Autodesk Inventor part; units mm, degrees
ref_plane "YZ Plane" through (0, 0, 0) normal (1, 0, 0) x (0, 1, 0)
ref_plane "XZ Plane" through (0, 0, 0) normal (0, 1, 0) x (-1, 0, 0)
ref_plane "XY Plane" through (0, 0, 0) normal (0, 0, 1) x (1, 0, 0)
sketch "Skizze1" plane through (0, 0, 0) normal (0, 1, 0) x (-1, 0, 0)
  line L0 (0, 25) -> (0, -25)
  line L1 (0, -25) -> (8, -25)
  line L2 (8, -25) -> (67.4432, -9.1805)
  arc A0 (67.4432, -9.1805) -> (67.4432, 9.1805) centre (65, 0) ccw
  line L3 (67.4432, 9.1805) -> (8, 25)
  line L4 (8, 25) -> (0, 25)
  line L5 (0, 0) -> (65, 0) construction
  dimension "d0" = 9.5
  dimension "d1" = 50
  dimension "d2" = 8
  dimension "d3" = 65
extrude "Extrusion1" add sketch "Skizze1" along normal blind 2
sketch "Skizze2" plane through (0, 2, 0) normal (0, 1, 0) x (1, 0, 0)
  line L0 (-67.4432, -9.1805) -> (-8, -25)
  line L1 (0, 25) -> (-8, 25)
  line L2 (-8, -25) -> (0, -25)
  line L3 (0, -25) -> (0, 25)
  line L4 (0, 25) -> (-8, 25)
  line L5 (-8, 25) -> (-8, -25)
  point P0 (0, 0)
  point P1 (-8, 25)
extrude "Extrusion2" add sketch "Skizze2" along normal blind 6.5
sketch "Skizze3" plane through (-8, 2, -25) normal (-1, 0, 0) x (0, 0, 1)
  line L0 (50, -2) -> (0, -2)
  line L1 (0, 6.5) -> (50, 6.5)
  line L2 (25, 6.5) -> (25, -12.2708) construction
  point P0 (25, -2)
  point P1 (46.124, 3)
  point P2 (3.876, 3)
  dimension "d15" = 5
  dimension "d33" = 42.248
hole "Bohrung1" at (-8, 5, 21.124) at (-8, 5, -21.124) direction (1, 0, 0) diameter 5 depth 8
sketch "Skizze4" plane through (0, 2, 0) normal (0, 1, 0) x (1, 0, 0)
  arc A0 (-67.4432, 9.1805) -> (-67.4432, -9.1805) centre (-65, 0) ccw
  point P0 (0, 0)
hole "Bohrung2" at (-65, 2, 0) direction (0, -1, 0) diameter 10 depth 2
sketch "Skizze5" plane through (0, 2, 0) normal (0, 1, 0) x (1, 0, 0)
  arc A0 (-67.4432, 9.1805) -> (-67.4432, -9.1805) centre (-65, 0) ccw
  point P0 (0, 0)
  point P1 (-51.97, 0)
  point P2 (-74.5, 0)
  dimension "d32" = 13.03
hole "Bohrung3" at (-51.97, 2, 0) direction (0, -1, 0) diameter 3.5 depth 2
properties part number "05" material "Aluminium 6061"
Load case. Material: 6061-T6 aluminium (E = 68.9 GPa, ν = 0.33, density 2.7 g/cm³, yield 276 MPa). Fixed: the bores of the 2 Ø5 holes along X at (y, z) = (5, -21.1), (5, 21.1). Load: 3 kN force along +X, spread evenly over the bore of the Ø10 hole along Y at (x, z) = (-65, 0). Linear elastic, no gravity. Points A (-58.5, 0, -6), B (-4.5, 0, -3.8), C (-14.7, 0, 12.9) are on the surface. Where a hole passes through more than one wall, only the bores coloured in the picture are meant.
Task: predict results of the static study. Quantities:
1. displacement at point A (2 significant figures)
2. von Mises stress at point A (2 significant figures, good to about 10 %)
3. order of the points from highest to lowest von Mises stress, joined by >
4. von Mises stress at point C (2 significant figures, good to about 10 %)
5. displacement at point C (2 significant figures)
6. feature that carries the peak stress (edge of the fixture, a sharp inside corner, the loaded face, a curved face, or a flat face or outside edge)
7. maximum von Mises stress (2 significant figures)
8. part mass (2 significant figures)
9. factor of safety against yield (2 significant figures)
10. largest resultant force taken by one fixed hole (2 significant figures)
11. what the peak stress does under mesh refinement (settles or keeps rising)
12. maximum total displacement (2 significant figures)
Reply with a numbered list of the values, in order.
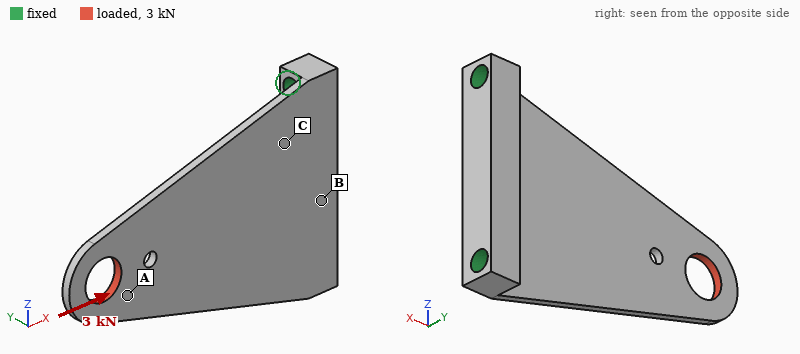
1. 0.090 mm
2. 83 MPa
3. A > C > B
4. 40 MPa
5. 0.019 mm
6. the loaded face
7. 200 MPa
8. 19 g
9. 1.4
10. 1.6 kN
11. settles
12. 0.12 mm
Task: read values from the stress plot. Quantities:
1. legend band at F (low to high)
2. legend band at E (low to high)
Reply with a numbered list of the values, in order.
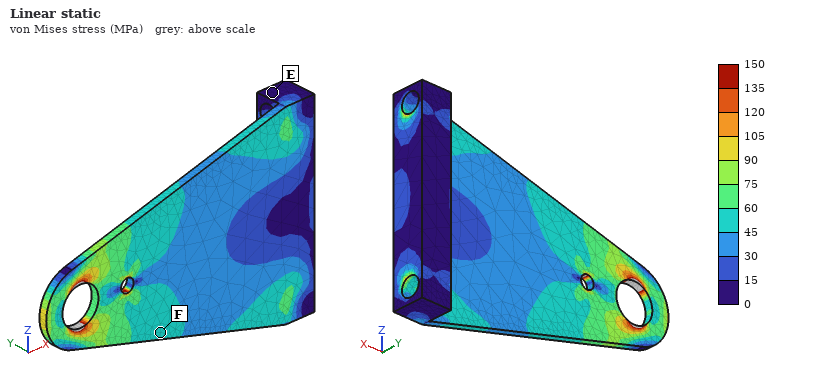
1. 45 to 60 MPa
2. 0 to 15 MPa
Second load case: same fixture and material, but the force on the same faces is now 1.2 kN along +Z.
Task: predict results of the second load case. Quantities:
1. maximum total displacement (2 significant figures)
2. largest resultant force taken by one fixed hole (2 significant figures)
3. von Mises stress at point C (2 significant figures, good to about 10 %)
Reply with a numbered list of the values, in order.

1. 0.21 mm
2. 1.9 kN
3. 44 MPa
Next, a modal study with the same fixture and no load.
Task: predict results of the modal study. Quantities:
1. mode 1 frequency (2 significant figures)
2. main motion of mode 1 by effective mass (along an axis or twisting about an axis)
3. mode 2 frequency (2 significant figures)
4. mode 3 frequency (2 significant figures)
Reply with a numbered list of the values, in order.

1. 570 Hz
2. along Y
3. 2500 Hz
4. 2600 Hz
